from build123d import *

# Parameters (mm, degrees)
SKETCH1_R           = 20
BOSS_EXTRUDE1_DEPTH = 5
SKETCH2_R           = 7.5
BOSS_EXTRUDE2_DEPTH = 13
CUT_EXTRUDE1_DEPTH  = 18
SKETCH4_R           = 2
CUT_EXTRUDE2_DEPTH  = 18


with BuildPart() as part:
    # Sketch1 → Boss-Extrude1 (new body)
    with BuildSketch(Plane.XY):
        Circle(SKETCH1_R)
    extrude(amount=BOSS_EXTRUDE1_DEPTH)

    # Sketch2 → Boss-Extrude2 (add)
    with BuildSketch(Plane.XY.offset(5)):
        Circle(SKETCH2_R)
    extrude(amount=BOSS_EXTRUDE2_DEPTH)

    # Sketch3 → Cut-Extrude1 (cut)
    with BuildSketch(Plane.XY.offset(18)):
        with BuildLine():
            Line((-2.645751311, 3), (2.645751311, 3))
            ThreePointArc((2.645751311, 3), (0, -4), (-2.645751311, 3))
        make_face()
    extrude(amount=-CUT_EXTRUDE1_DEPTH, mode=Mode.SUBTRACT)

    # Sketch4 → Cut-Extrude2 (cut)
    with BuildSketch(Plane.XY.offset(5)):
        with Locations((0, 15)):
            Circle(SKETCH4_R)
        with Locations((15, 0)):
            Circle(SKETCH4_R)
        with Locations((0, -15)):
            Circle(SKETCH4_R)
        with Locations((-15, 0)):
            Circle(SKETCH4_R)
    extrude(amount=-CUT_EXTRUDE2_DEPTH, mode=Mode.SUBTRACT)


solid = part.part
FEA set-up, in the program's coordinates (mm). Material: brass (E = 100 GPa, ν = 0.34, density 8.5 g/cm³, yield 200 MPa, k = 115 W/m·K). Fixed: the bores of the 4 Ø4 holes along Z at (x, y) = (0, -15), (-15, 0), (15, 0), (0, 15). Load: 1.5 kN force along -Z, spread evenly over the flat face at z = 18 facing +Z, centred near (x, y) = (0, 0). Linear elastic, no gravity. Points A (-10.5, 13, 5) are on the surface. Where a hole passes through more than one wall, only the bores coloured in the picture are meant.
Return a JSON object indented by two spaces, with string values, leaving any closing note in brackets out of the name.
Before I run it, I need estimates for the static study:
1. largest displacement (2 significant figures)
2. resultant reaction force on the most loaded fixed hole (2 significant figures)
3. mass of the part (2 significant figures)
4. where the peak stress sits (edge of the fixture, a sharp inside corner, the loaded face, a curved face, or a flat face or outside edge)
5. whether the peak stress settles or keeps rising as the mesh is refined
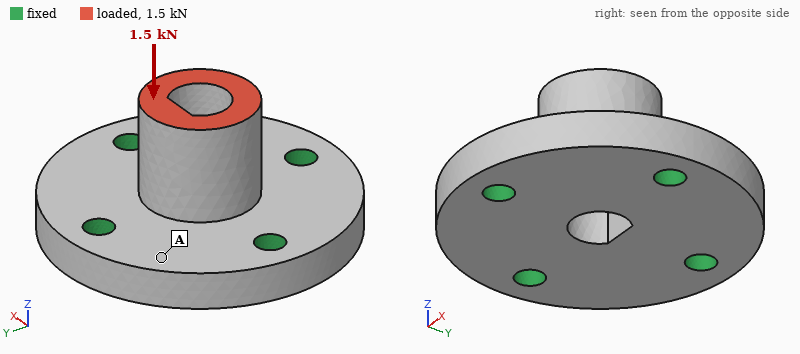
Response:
{
  "largest displacement": "4.9 µm",
  "resultant reaction force on the most loaded fixed hole": "400 N",
  "mass of the part": "64 g",
  "where the peak stress sits": "edge of the fixture",
  "whether the peak stress settles or keeps rising as the mesh is refined": "keeps rising"
}
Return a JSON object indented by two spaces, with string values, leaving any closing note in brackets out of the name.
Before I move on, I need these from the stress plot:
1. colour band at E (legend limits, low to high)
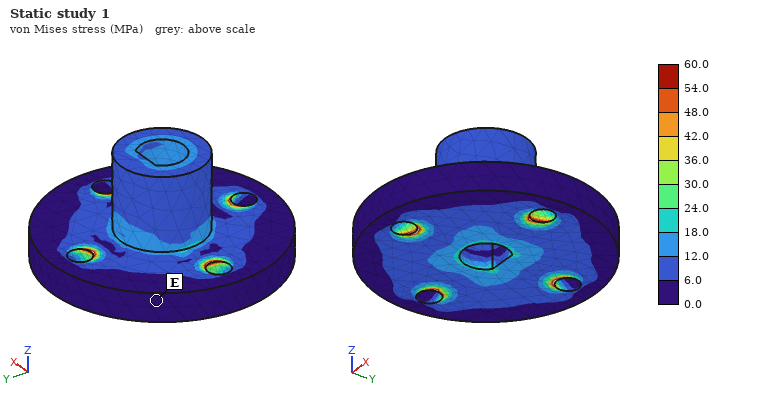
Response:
{
  "colour band at E": "0.0 to 6.0 MPa"
}
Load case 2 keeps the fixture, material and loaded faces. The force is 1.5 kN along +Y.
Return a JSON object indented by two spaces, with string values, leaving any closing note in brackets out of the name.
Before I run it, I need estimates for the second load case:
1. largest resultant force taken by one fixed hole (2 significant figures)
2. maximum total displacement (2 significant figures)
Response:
{
  "largest resultant force taken by one fixed hole": "1.0 kN",
  "maximum total displacement": "28 µm"
}
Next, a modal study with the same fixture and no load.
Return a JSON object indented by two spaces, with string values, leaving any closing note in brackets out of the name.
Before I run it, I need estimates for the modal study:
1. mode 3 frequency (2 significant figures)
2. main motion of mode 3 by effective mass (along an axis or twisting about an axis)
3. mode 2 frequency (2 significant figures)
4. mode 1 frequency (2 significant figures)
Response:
{
  "mode 3 frequency": "20 kHz",
  "main motion of mode 3 by effective mass": "along Z",
  "mode 2 frequency": "16 kHz",
  "mode 1 frequency": "16 kHz"
}
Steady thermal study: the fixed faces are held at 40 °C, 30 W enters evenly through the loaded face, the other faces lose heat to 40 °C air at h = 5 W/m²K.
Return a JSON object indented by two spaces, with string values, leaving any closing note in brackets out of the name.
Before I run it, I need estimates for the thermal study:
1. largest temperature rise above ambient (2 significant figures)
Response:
{
  "largest temperature rise above ambient": "36 K"
}
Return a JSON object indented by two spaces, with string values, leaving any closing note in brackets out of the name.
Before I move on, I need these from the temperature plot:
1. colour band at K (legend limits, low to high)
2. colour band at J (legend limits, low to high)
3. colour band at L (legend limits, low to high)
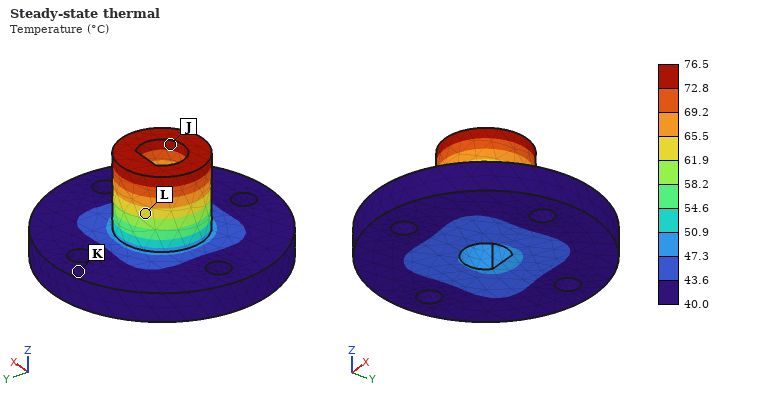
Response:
{
  "colour band at K": "40.0 to 43.6 °C",
  "colour band at J": "72.8 to 76.5 °C",
  "colour band at L": "61.9 to 65.5 °C"
}
